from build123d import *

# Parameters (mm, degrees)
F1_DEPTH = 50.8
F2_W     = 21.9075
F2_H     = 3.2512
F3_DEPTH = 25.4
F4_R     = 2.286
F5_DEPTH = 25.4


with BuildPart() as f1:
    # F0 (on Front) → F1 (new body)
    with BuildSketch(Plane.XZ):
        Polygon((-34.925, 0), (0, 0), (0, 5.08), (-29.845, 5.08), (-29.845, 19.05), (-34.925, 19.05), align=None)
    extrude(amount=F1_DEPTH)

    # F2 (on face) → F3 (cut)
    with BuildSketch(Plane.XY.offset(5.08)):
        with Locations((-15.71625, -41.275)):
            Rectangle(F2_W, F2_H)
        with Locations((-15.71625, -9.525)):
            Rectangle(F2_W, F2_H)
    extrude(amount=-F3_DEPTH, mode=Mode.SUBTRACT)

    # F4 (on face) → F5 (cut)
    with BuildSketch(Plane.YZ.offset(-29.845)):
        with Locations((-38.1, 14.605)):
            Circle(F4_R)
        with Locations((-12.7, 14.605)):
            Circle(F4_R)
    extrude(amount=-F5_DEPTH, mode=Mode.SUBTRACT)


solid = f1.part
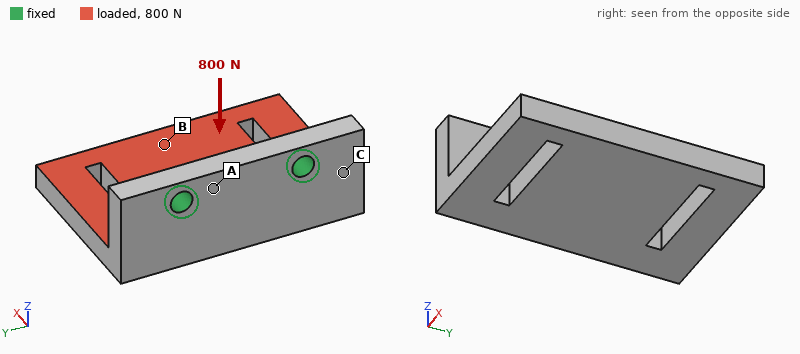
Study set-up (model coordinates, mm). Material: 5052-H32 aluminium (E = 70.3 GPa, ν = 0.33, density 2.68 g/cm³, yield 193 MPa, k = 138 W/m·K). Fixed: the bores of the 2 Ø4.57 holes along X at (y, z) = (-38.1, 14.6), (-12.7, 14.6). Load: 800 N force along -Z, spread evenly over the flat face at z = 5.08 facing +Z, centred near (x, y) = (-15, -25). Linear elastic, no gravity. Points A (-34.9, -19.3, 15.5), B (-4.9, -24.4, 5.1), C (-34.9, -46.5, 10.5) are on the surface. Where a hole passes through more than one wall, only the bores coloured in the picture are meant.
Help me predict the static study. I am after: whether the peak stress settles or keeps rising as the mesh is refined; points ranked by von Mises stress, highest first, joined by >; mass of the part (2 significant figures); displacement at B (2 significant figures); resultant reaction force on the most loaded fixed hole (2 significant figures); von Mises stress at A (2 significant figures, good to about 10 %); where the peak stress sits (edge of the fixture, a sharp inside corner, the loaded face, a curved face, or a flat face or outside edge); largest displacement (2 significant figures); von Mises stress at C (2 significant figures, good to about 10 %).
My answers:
keeps rising
C > A > B
31 g
0.19 mm
400 N
24 MPa
edge of the fixture
0.24 mm
46 MPa
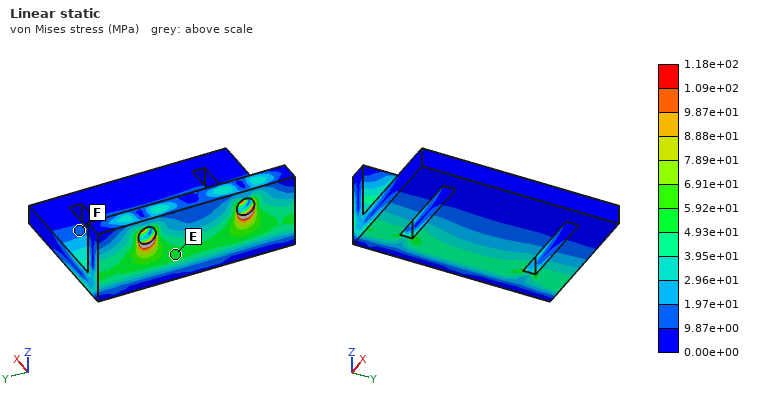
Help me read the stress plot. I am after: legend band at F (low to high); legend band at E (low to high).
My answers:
9.87e+00 to 1.97e+01 MPa
4.93e+01 to 5.92e+01 MPa
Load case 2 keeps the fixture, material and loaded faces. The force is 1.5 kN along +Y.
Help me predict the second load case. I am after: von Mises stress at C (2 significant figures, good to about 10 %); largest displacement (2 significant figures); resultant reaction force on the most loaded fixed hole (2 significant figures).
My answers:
27 MPa
0.10 mm
1.2 kN
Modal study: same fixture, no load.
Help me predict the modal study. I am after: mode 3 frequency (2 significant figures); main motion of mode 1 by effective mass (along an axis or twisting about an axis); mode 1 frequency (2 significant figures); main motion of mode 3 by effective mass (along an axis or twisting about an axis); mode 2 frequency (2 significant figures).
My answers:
7000 Hz
along Z
2600 Hz
along Y
4900 Hz
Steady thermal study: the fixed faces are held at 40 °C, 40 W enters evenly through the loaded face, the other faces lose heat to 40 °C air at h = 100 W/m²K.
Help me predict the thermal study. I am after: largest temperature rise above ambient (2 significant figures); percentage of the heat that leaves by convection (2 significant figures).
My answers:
30 K
19 %
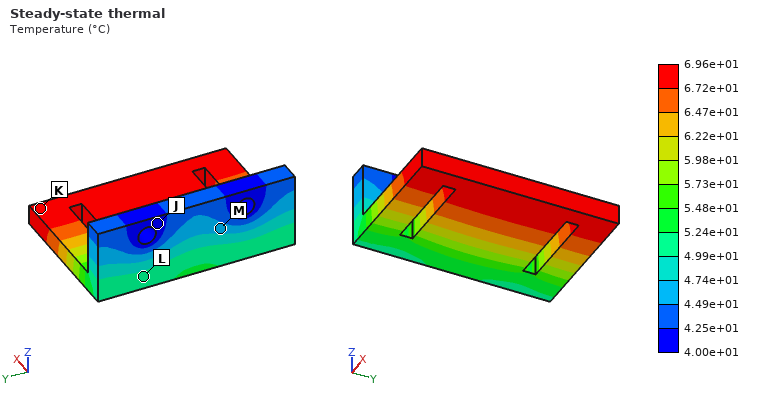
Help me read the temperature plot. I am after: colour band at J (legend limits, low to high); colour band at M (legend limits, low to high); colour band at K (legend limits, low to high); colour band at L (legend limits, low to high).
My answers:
4.00e+01 to 4.25e+01 °C
4.49e+01 to 4.74e+01 °C
6.72e+01 to 6.96e+01 °C
4.99e+01 to 5.24e+01 °C
